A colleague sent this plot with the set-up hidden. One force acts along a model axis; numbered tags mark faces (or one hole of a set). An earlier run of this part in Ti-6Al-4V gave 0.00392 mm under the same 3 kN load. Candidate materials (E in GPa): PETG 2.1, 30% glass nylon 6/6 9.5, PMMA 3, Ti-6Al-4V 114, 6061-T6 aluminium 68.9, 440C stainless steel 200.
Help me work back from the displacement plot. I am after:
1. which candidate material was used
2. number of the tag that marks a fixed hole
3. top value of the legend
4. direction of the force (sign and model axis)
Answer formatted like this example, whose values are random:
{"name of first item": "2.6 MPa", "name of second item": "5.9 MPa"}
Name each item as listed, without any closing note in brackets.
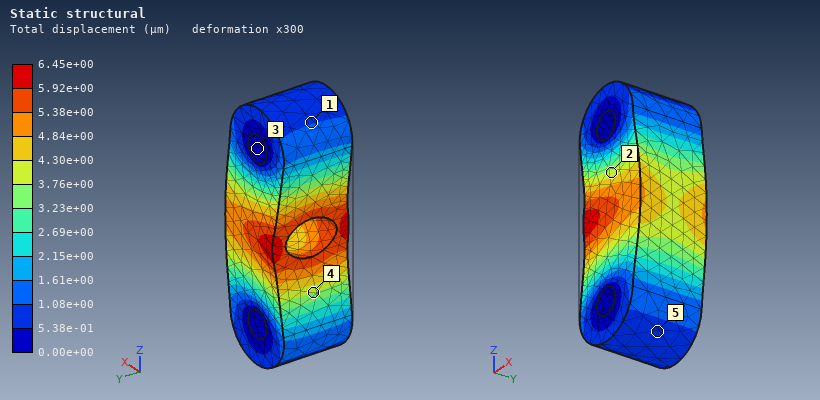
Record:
{"which candidate material was used": "6061-T6 aluminium", "number of the tag that marks a fixed hole": "3", "top value of the legend": "6.45e+00 µm", "direction of the force": "+X"}
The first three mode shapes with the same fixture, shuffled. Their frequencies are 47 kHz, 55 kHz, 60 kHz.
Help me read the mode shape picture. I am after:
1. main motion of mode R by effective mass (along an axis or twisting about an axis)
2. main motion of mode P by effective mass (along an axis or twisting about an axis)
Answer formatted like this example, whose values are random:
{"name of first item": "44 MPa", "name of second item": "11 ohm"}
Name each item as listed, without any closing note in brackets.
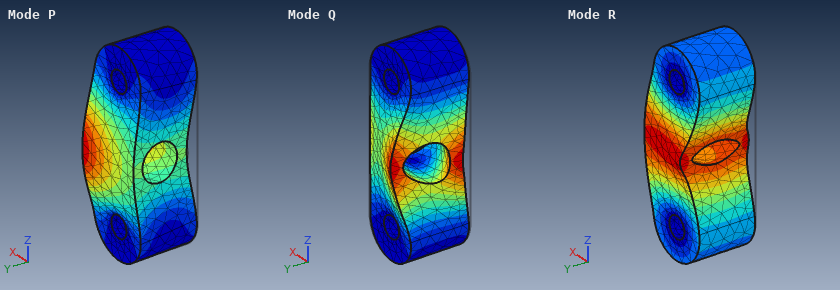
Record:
{"main motion of mode R by effective mass": "along X", "main motion of mode P by effective mass": "along Y"}
